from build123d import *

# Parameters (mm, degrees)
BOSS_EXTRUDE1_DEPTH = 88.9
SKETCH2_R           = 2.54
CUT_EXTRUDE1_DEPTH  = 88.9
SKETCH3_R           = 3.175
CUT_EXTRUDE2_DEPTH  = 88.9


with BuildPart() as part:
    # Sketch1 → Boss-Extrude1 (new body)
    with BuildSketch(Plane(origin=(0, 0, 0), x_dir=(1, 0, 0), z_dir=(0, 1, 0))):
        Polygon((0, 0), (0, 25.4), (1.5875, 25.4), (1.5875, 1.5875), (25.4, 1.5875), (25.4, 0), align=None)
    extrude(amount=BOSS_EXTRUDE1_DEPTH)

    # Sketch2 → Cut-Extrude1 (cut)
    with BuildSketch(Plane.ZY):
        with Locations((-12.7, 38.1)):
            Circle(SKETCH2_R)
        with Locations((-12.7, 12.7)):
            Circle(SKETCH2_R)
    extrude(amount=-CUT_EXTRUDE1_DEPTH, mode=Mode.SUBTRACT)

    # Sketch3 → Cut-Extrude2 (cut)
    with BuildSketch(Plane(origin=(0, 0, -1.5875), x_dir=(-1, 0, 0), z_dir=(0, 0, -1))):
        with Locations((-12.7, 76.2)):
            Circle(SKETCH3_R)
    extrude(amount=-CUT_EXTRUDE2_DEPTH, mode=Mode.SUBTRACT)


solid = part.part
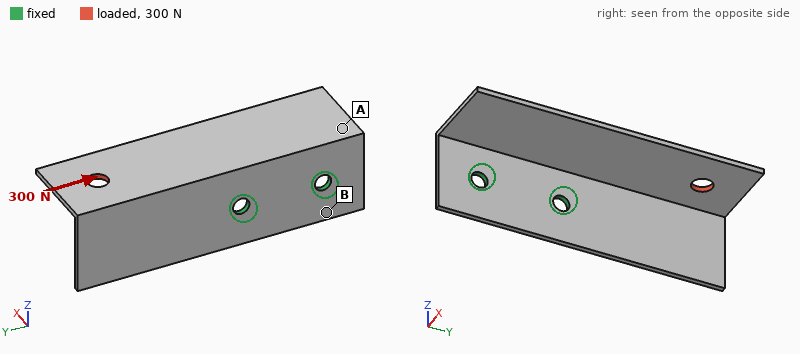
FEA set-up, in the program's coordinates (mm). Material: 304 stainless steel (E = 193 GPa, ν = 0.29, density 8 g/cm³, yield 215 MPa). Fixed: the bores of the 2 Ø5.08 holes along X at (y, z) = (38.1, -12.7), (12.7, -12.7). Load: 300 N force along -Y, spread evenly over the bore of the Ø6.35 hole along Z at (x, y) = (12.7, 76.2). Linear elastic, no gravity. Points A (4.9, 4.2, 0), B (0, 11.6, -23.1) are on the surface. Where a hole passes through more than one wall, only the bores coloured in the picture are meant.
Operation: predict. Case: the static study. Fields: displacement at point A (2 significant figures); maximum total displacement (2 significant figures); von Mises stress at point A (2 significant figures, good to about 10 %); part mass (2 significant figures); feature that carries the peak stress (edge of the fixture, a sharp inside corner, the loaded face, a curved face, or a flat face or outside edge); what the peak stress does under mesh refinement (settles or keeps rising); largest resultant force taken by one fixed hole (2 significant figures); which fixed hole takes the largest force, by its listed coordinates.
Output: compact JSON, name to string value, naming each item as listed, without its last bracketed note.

{"displacement at point A": "0.035 mm", "maximum total displacement": "0.11 mm", "von Mises stress at point A": "24 MPa", "part mass": "55 g", "feature that carries the peak stress": "edge of the fixture", "what the peak stress does under mesh refinement": "keeps rising", "largest resultant force taken by one fixed hole": "230 N", "which fixed hole takes the largest force, by its listed coordinates": "(38.1, -12.7)"}
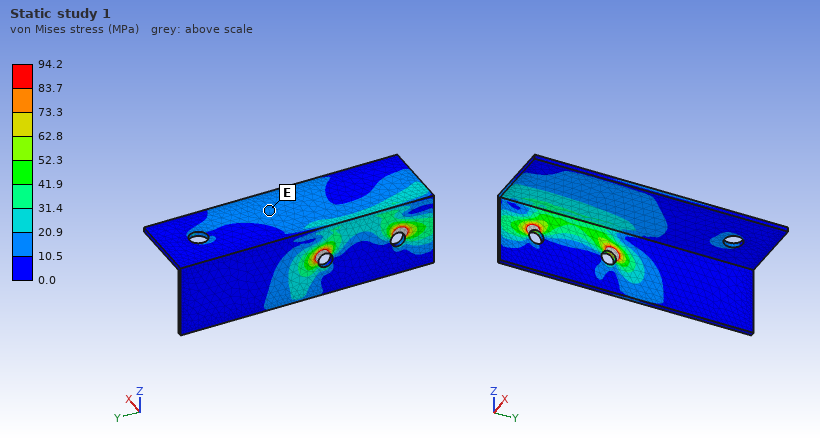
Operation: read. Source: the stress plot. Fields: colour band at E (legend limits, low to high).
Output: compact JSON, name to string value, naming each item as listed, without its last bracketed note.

{"colour band at E": "10.5 to 20.9 MPa"}
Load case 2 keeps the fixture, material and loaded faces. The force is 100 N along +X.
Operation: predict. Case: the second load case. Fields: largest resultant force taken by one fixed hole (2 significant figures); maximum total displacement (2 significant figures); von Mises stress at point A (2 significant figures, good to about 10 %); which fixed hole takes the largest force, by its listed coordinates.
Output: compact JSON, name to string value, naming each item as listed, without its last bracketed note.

{"largest resultant force taken by one fixed hole": "220 N", "maximum total displacement": "0.19 mm", "von Mises stress at point A": "35 MPa", "which fixed hole takes the largest force, by its listed coordinates": "(38.1, -12.7)"}
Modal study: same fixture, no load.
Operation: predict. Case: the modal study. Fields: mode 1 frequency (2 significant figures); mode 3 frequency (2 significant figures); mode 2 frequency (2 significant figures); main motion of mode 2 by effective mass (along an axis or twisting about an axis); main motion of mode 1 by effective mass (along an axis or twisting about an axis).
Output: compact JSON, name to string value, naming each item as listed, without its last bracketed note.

{"mode 1 frequency": "910 Hz", "mode 3 frequency": "1500 Hz", "mode 2 frequency": "1100 Hz", "main motion of mode 2 by effective mass": "along X", "main motion of mode 1 by effective mass": "along Z"}
